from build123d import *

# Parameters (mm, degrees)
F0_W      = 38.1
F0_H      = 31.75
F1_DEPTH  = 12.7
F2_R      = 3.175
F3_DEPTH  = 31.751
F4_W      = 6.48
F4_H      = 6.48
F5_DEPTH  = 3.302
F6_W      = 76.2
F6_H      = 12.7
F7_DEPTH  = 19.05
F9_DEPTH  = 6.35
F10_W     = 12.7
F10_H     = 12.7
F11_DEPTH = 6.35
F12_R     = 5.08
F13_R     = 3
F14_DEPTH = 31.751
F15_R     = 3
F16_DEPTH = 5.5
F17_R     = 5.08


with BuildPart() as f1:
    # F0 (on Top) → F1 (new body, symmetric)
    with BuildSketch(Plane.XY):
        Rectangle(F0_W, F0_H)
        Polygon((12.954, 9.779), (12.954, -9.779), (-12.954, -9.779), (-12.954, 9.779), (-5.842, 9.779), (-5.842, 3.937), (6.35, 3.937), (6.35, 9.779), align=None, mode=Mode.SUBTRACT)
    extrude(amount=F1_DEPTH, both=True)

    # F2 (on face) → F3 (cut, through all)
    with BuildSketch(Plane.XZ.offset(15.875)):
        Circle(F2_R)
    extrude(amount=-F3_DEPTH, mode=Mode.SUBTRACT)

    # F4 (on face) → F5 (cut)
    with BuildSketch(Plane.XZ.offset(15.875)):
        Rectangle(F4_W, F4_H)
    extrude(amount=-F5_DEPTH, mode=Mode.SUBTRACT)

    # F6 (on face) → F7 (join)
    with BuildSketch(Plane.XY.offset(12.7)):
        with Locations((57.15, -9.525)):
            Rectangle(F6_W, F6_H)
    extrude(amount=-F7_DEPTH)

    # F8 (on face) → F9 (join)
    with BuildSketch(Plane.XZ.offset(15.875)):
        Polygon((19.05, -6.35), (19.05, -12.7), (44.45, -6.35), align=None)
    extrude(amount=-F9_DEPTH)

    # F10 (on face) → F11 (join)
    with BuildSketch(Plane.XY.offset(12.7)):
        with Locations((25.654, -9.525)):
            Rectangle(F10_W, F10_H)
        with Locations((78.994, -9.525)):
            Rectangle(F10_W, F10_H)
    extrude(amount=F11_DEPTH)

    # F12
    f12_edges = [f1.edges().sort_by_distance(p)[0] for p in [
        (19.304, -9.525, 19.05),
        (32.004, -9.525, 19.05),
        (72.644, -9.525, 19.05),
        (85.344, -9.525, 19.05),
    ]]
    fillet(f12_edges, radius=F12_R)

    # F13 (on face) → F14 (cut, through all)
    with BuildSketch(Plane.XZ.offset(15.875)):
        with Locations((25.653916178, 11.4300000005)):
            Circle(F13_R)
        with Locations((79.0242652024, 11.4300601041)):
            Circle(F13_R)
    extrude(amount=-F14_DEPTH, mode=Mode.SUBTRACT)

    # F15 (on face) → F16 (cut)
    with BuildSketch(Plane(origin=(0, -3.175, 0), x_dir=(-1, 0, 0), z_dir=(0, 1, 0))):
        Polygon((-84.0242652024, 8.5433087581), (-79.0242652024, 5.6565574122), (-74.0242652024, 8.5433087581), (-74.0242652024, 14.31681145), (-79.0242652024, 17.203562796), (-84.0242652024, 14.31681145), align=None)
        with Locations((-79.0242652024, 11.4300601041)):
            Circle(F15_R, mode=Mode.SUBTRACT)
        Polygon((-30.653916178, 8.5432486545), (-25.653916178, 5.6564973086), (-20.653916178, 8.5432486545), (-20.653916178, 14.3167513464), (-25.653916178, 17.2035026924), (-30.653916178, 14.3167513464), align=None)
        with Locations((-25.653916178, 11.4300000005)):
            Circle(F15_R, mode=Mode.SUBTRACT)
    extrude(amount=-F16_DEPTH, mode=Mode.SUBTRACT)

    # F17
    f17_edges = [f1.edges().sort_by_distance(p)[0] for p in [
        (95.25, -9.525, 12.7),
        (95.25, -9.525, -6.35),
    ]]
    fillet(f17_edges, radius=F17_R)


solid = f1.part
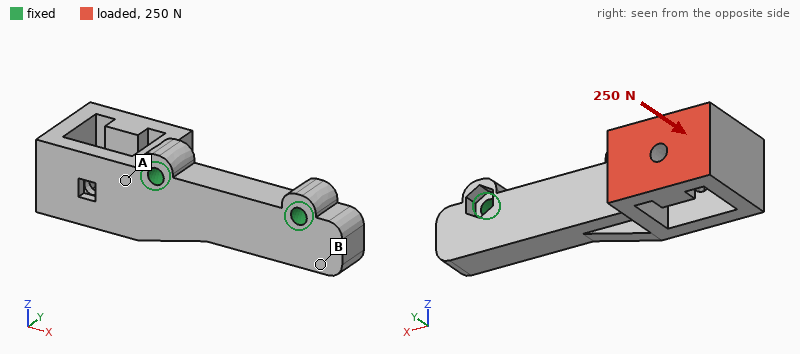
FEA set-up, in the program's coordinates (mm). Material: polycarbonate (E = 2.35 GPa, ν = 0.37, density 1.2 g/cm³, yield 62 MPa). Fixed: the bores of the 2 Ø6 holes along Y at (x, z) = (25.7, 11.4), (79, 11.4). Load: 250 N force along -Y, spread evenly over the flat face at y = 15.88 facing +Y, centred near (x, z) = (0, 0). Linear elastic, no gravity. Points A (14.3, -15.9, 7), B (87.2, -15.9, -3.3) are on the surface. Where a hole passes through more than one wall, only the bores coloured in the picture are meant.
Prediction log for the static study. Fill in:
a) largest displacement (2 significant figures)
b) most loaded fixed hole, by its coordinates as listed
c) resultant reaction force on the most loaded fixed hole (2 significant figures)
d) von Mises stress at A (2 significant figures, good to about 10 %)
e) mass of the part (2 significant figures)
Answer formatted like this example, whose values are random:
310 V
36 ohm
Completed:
1.3 mm
(25.7, 11.4)
330 N
9.8 MPa
46 g
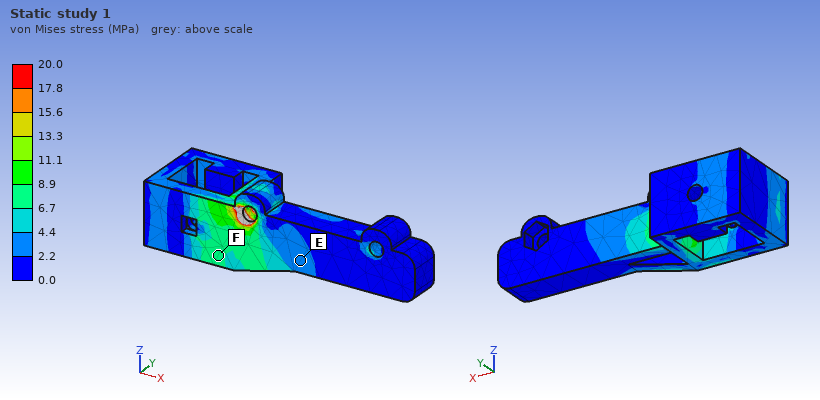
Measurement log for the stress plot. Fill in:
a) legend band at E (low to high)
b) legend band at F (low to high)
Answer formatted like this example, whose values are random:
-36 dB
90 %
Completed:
2.2 to 4.4 MPa
6.7 to 8.9 MPa
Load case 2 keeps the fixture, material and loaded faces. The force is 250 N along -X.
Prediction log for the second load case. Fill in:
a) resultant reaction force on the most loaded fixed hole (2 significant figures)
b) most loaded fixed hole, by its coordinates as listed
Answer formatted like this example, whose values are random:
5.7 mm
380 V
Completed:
200 N
(79, 11.4)
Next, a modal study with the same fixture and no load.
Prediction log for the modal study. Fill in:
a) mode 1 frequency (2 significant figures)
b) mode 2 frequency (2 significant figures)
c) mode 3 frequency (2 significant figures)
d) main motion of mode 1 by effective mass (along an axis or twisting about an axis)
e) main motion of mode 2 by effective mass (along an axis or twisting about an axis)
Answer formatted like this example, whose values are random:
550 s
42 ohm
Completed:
530 Hz
790 Hz
1500 Hz
along Y
along Z
